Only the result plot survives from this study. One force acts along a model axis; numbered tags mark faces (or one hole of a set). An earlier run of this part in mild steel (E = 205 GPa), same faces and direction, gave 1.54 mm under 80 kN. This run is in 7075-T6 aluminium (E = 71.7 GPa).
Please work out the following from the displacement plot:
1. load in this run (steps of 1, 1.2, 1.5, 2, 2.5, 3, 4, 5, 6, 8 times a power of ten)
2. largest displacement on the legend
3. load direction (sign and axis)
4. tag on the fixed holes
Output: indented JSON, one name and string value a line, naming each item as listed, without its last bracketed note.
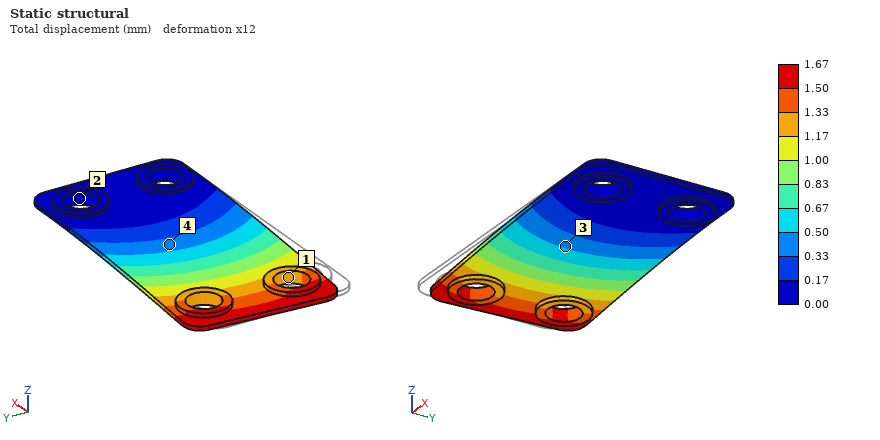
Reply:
{
  "load in this run": "30 kN",
  "largest displacement on the legend": "1.67 mm",
  "load direction": "+Y",
  "tag on the fixed holes": "2"
}
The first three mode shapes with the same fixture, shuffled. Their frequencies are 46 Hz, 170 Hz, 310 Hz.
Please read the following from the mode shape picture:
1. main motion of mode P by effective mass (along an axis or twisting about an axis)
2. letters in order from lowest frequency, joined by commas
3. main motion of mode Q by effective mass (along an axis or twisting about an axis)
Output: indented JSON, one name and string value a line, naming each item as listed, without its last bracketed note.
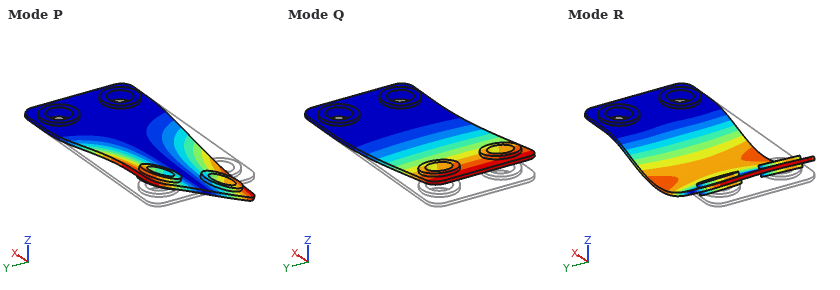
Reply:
{
  "main motion of mode P by effective mass": "twisting about X",
  "letters in order from lowest frequency, joined by commas": "Q, P, R",
  "main motion of mode Q by effective mass": "along Z"
}
